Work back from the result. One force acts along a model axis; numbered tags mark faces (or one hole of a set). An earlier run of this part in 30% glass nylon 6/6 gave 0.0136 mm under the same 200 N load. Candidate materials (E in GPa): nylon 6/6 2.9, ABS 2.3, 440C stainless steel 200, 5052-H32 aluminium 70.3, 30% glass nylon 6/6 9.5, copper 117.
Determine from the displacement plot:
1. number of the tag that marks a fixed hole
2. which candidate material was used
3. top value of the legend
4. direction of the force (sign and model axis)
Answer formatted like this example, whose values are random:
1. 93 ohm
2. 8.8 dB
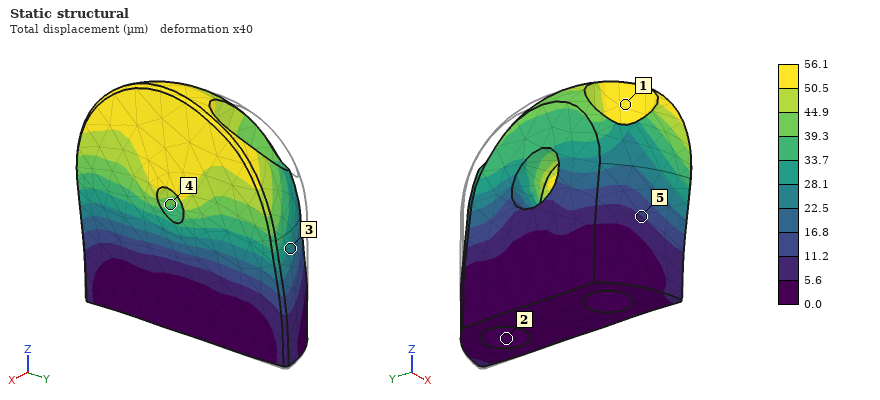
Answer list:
1. 2
2. ABS
3. 56.1 µm
4. -Y
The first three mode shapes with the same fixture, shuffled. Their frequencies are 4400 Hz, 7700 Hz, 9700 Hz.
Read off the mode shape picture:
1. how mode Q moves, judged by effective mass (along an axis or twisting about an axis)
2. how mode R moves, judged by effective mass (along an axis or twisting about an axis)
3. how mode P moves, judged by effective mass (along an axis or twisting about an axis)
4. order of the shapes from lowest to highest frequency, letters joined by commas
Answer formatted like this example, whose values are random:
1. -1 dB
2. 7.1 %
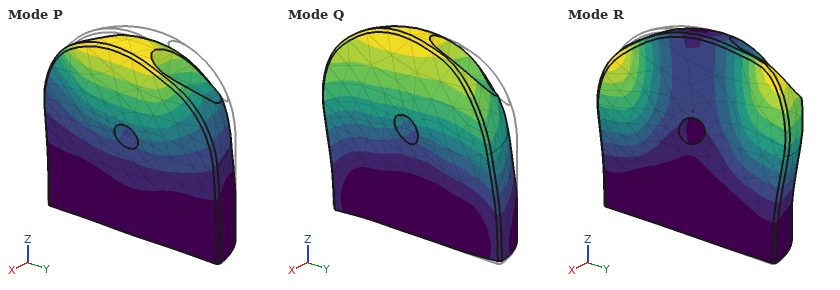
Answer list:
1. along Y
2. twisting about Z
3. along X
4. P, Q, R
